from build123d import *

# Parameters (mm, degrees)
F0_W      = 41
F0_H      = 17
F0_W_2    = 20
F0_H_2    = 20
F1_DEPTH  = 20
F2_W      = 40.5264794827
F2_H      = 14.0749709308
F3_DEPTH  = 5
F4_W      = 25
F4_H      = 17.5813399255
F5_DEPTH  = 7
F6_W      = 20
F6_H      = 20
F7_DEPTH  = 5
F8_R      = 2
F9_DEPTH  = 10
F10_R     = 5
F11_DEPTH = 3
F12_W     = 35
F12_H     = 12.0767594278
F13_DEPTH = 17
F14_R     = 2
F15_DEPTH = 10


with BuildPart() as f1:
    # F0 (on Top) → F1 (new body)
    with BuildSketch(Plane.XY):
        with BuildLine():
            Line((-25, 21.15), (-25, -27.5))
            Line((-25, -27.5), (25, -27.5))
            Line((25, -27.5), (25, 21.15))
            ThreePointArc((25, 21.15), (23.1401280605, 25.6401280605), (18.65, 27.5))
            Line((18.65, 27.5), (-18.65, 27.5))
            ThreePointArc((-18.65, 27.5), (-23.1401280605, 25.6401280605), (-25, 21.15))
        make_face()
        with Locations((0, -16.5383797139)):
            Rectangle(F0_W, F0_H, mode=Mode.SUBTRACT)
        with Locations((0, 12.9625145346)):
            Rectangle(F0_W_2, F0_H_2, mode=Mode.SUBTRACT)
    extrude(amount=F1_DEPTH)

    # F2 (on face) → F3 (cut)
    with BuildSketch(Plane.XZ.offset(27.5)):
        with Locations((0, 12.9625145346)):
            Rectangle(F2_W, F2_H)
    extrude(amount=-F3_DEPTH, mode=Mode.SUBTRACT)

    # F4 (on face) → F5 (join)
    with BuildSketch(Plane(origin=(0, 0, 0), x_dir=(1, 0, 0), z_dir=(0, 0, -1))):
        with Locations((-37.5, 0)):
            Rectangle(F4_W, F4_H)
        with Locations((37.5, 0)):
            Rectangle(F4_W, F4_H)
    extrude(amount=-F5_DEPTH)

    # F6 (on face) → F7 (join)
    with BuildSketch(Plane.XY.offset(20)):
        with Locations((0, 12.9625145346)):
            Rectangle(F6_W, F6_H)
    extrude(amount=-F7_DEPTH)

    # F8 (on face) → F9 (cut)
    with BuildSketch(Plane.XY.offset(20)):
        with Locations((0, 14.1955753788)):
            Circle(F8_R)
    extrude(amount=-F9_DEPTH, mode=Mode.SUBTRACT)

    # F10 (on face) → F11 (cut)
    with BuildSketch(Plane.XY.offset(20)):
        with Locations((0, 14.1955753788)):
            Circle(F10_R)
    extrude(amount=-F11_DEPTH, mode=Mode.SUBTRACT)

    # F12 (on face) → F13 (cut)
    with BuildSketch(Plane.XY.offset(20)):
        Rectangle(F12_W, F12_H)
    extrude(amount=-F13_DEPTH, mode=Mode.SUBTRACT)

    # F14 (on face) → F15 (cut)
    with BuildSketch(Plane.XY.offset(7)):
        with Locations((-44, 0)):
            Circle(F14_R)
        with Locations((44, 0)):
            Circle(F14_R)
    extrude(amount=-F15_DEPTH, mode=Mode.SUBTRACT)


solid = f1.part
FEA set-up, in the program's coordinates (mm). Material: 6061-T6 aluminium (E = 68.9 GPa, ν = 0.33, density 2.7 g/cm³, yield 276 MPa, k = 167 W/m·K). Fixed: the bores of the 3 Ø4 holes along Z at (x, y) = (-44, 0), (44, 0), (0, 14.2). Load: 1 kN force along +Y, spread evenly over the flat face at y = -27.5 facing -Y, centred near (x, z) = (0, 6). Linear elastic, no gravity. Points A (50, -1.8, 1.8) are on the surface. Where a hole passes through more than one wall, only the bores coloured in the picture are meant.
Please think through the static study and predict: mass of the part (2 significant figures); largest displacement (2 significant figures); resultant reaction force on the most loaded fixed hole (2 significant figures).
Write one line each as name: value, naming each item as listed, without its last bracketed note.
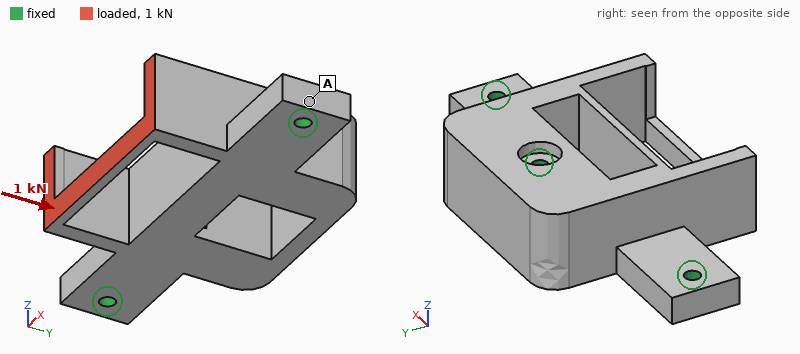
mass of the part: 88 g
largest displacement: 0.28 mm
resultant reaction force on the most loaded fixed hole: 400 N
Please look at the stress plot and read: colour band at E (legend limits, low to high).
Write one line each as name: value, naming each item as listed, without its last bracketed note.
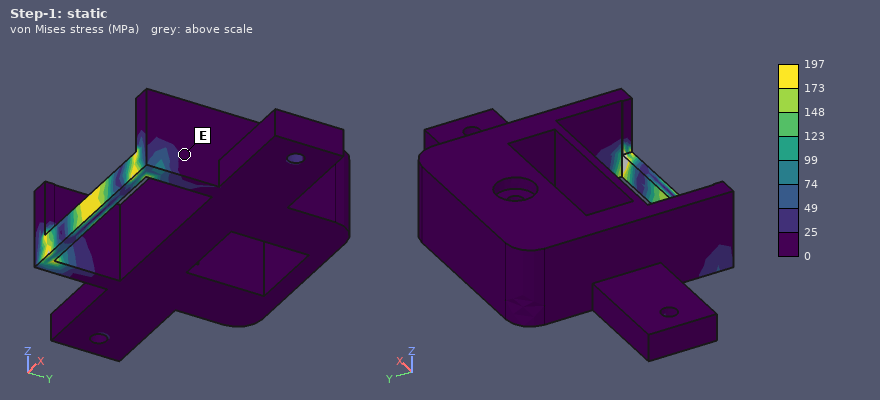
colour band at E: 0 to 25 MPa
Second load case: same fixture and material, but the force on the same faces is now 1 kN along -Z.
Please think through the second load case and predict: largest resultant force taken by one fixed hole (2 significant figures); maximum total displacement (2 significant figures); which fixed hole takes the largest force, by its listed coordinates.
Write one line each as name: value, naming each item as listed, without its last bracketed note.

largest resultant force taken by one fixed hole: 1.3 kN
maximum total displacement: 0.20 mm
which fixed hole takes the largest force, by its listed coordinates: (0, 14.2)
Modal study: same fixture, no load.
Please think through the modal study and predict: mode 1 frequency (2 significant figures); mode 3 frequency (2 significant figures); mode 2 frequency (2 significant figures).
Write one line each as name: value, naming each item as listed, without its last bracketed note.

mode 1 frequency: 4700 Hz
mode 3 frequency: 6400 Hz
mode 2 frequency: 6400 Hz
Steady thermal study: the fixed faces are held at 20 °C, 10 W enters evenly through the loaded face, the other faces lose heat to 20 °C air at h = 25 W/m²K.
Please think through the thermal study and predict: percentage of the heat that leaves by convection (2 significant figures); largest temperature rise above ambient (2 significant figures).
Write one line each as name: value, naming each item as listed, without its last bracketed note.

percentage of the heat that leaves by convection: 12 %
largest temperature rise above ambient: 24 K
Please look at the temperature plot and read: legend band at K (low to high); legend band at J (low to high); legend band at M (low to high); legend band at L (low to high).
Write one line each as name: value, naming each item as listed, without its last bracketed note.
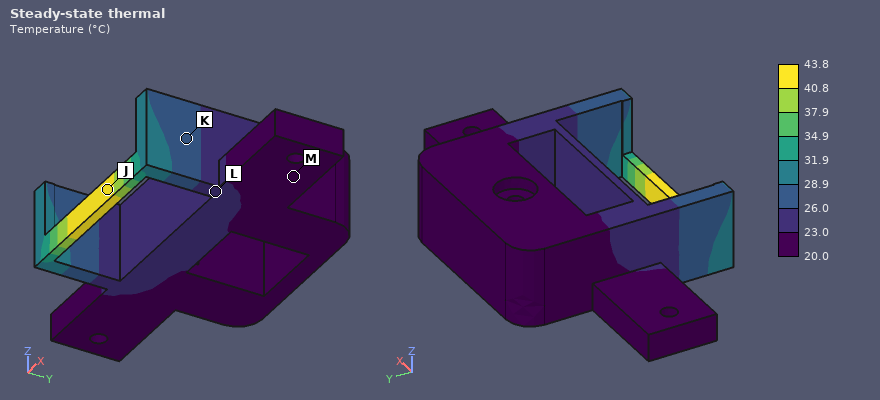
legend band at K: 26.0 to 28.9 °C
legend band at J: 40.8 to 43.8 °C
legend band at M: 20.0 to 23.0 °C
legend band at L: 23.0 to 26.0 °C
